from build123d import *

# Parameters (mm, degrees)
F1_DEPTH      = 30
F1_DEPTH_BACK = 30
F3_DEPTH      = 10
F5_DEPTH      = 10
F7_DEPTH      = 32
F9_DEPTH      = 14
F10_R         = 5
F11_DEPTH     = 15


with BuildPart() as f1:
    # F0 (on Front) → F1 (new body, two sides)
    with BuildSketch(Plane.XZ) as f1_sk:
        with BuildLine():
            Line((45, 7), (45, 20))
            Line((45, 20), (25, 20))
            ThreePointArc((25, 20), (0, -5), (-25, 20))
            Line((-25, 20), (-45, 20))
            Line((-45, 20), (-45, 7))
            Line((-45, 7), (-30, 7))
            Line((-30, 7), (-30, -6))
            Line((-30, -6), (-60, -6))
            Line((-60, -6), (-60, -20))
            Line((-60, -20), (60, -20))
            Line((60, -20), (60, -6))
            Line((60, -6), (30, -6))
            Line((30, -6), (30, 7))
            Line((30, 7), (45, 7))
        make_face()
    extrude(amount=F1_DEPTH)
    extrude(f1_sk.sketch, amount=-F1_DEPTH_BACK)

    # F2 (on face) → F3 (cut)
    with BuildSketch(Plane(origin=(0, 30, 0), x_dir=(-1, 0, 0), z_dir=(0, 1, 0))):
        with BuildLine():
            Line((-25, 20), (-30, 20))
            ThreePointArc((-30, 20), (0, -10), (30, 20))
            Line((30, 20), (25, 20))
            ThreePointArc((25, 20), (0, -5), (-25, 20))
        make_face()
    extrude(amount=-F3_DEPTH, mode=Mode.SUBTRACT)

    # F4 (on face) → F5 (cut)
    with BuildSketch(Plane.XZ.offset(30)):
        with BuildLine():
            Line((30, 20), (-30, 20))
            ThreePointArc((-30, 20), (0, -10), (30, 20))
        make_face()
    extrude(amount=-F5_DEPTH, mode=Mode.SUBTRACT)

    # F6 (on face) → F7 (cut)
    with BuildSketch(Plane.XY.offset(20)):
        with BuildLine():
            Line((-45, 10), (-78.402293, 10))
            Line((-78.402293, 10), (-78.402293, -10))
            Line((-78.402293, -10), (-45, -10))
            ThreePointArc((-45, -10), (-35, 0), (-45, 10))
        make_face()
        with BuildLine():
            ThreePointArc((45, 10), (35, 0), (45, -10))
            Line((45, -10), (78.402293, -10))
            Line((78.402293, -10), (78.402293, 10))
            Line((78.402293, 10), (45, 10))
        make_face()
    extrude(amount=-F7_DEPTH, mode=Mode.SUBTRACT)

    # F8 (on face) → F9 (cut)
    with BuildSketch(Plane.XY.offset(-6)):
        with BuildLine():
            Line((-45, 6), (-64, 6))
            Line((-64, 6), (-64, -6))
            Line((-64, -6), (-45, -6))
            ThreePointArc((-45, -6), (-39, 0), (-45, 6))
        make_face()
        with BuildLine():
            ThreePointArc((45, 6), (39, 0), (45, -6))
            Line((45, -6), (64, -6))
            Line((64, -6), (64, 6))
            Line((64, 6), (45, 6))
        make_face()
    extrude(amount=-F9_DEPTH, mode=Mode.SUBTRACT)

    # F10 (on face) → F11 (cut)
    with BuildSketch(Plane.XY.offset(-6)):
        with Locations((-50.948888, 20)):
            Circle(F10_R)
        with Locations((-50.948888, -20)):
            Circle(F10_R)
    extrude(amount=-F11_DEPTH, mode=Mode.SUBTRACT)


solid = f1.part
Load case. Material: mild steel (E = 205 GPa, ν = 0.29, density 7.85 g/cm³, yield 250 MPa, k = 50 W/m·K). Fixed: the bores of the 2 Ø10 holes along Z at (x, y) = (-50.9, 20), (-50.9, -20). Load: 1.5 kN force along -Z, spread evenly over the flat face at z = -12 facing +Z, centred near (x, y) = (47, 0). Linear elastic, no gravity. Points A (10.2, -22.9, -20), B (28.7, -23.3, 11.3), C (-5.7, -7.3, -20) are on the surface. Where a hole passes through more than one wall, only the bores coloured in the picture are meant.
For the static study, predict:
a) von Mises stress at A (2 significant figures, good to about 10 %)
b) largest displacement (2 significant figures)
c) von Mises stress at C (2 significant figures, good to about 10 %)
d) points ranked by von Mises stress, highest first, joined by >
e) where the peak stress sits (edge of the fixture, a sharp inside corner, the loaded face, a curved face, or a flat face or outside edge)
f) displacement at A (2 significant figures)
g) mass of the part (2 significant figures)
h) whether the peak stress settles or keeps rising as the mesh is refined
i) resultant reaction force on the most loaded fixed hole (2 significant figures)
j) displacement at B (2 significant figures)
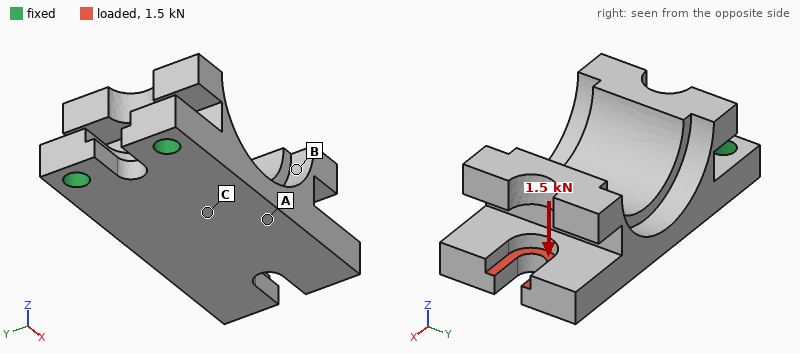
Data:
21 MPa
0.18 mm
35 MPa
C > A > B
edge of the fixture
0.075 mm
1.1 kg
keeps rising
750 N
0.12 mm
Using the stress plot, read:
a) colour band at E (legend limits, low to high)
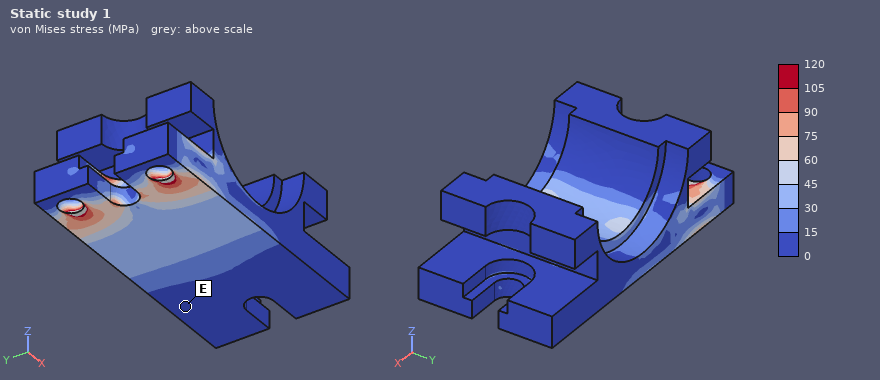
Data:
0 to 15 MPa
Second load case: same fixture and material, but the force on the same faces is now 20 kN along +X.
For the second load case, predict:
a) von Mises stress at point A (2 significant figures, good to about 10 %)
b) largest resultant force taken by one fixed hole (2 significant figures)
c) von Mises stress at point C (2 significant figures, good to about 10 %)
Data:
18 MPa
10 kN
18 MPa
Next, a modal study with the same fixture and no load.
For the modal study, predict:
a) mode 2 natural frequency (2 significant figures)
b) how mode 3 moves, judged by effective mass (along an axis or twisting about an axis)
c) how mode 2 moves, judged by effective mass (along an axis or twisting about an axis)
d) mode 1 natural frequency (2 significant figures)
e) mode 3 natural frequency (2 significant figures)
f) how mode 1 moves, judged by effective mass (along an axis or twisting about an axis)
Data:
2700 Hz
along Y
along Y
840 Hz
3300 Hz
along Z
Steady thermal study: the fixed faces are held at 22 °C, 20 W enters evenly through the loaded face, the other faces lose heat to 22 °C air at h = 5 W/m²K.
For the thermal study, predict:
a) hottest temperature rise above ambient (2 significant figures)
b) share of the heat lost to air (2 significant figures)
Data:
49 K
15 %
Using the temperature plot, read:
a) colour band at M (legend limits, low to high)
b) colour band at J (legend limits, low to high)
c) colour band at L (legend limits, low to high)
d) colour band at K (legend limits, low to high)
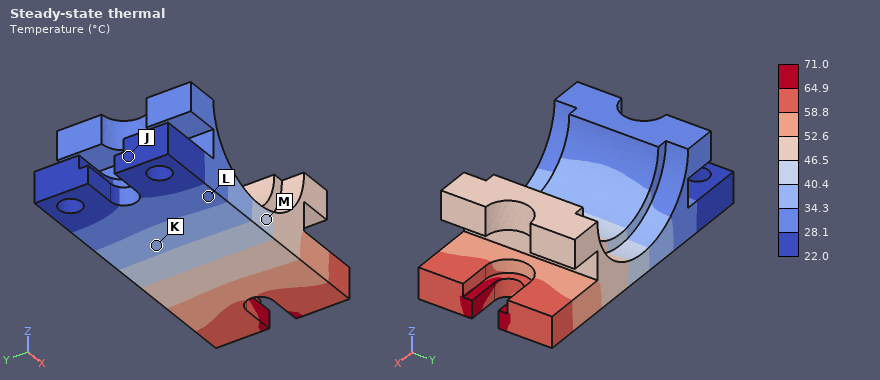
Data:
40.4 to 46.5 °C
22.0 to 28.1 °C
28.1 to 34.3 °C
34.3 to 40.4 °C
